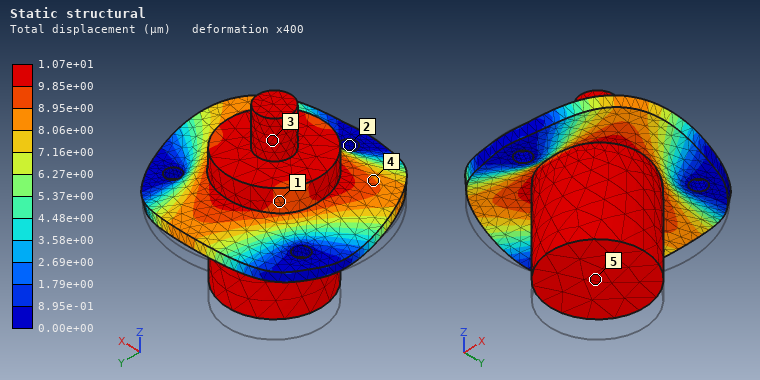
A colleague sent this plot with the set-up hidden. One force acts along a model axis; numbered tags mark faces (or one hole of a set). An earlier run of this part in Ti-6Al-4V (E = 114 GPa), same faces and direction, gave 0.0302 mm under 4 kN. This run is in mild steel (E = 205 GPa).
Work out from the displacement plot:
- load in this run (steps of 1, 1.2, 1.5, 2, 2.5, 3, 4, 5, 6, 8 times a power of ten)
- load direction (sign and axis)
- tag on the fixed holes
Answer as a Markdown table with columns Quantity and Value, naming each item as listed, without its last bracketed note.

| Quantity | Value |
|---|---|
| load in this run | 2.5 kN |
| load direction | +Z |
| tag on the fixed holes | 2 |
